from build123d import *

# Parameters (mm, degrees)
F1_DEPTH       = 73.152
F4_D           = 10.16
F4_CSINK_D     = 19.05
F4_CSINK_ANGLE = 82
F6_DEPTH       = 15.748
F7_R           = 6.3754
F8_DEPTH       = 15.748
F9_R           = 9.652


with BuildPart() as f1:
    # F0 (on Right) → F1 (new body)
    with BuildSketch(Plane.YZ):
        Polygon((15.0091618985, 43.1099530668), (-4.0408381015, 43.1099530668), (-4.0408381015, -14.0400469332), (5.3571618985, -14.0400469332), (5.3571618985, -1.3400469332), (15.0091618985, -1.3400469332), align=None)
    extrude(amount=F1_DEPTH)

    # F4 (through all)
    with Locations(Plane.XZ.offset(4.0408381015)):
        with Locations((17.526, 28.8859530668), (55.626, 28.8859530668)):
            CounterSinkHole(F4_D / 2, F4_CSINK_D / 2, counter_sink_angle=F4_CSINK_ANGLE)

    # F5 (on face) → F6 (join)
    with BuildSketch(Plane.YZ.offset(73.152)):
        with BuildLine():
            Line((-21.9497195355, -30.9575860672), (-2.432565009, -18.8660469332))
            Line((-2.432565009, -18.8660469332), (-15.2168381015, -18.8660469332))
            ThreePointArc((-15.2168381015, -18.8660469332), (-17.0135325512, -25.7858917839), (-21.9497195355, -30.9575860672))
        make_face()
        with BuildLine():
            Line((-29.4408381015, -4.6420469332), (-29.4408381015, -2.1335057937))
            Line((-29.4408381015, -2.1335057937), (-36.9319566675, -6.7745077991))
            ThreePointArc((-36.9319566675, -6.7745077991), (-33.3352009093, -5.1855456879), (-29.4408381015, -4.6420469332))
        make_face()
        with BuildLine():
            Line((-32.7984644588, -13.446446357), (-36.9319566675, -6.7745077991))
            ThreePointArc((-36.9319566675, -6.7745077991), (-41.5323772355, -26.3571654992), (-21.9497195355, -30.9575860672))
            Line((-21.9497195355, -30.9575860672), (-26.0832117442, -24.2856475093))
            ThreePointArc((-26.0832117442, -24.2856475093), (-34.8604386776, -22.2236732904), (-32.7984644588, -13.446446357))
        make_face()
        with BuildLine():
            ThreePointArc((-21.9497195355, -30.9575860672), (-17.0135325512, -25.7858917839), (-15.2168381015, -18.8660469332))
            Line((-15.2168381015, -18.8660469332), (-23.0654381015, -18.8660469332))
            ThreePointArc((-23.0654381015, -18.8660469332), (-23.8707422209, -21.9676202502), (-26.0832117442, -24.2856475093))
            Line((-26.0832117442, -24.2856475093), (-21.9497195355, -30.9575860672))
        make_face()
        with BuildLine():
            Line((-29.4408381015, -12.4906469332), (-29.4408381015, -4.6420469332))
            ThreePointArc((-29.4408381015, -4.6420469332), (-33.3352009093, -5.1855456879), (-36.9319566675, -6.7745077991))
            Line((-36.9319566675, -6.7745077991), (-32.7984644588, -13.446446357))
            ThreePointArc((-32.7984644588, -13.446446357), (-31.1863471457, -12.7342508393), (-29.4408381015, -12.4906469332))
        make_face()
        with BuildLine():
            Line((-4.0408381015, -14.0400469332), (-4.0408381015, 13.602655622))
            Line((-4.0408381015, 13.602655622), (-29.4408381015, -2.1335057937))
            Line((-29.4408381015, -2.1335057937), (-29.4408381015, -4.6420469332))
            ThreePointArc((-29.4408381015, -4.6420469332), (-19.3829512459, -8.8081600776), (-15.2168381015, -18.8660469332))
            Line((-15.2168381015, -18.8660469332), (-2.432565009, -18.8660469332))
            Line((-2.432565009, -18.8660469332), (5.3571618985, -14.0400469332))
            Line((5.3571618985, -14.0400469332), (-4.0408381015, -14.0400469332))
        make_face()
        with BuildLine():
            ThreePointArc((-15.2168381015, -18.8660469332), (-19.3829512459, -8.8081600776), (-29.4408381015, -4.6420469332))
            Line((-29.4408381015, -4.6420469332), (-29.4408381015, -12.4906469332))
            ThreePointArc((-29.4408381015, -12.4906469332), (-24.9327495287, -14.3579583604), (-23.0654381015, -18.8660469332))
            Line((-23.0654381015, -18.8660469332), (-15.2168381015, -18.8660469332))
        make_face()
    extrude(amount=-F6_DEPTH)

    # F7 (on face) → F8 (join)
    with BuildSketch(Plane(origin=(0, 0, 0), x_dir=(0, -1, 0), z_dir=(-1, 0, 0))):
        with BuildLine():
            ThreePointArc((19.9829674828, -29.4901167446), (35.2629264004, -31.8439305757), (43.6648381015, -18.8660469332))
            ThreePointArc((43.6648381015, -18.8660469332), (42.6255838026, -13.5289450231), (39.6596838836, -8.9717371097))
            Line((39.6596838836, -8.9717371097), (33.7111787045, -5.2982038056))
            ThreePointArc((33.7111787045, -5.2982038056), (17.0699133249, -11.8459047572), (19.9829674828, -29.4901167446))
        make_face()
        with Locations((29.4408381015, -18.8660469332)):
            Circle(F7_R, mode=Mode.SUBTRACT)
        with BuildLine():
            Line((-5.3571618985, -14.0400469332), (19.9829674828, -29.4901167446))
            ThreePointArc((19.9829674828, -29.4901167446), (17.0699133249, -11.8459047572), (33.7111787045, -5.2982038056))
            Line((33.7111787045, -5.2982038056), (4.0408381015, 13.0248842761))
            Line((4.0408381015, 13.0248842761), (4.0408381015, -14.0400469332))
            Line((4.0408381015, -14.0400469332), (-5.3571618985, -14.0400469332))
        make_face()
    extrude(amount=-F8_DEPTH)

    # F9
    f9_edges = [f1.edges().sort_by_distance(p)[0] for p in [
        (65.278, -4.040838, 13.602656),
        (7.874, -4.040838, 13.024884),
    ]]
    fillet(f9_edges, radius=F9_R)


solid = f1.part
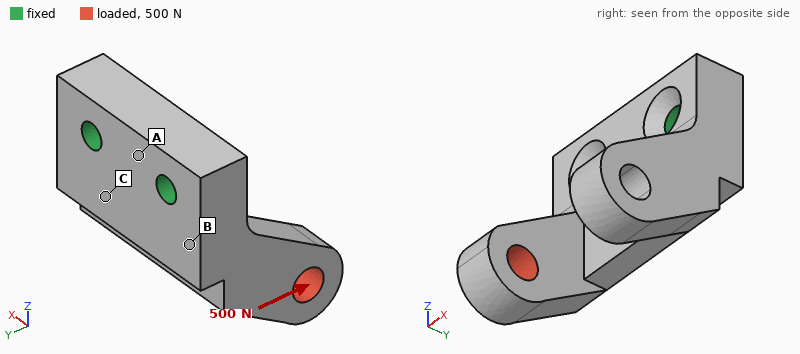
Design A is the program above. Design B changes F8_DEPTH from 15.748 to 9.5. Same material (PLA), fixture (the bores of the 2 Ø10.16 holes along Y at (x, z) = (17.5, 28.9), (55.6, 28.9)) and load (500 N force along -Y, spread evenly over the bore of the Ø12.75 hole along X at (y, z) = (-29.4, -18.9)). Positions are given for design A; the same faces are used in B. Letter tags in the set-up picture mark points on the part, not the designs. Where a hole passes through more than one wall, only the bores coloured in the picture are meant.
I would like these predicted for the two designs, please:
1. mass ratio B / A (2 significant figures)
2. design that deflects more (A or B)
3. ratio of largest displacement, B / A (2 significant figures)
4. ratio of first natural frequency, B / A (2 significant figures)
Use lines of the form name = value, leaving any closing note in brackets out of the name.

mass ratio B / A = 0.93
design that deflects more = B
ratio of largest displacement, B / A = 1.3
ratio of first natural frequency, B / A = 1.0
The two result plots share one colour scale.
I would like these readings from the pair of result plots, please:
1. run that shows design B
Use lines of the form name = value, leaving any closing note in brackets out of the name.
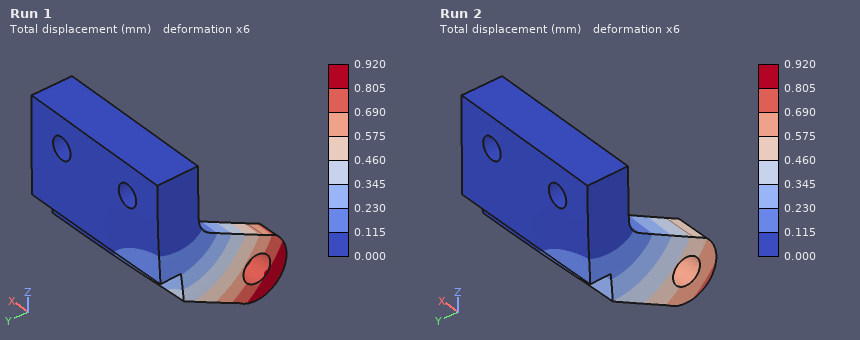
run that shows design B = Run 1
